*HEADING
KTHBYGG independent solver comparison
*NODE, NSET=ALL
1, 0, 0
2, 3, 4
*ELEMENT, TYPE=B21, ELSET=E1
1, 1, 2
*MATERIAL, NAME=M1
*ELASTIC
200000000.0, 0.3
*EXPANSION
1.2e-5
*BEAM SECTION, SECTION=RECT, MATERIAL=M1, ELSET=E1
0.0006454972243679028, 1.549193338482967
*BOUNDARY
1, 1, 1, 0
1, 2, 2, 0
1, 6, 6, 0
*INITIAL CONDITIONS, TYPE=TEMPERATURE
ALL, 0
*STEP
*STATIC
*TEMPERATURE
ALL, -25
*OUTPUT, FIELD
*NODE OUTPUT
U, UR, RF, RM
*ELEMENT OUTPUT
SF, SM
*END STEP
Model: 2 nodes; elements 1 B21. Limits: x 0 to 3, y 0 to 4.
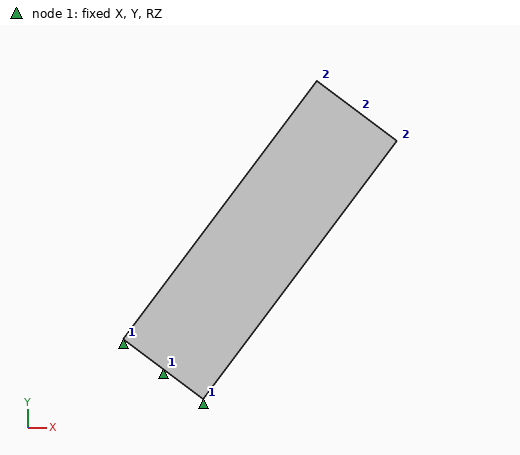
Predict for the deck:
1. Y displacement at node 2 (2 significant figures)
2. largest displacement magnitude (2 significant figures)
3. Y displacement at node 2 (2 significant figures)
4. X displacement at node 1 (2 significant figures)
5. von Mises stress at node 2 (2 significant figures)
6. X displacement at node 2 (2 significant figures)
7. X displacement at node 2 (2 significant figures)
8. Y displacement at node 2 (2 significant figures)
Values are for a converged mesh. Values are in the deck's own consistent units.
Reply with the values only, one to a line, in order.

-0.0013
0.0015
-0.0012
1.9e-04
0.0013
-0.0011
-9.0e-04
-0.0011
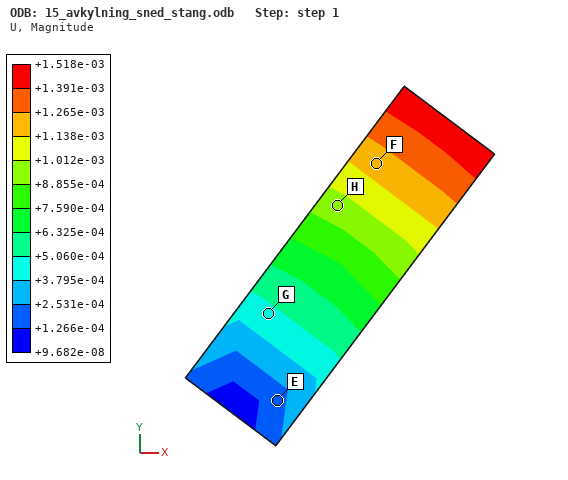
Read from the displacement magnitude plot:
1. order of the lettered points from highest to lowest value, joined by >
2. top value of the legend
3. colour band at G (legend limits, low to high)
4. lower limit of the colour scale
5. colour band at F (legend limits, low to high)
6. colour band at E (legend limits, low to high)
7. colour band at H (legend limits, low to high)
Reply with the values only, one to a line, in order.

F > H > G > E
+1.518e-03
+3.795e-04 to +5.060e-04
+9.682e-08
+1.138e-03 to +1.265e-03
+1.266e-04 to +2.531e-04
+8.855e-04 to +1.012e-03
